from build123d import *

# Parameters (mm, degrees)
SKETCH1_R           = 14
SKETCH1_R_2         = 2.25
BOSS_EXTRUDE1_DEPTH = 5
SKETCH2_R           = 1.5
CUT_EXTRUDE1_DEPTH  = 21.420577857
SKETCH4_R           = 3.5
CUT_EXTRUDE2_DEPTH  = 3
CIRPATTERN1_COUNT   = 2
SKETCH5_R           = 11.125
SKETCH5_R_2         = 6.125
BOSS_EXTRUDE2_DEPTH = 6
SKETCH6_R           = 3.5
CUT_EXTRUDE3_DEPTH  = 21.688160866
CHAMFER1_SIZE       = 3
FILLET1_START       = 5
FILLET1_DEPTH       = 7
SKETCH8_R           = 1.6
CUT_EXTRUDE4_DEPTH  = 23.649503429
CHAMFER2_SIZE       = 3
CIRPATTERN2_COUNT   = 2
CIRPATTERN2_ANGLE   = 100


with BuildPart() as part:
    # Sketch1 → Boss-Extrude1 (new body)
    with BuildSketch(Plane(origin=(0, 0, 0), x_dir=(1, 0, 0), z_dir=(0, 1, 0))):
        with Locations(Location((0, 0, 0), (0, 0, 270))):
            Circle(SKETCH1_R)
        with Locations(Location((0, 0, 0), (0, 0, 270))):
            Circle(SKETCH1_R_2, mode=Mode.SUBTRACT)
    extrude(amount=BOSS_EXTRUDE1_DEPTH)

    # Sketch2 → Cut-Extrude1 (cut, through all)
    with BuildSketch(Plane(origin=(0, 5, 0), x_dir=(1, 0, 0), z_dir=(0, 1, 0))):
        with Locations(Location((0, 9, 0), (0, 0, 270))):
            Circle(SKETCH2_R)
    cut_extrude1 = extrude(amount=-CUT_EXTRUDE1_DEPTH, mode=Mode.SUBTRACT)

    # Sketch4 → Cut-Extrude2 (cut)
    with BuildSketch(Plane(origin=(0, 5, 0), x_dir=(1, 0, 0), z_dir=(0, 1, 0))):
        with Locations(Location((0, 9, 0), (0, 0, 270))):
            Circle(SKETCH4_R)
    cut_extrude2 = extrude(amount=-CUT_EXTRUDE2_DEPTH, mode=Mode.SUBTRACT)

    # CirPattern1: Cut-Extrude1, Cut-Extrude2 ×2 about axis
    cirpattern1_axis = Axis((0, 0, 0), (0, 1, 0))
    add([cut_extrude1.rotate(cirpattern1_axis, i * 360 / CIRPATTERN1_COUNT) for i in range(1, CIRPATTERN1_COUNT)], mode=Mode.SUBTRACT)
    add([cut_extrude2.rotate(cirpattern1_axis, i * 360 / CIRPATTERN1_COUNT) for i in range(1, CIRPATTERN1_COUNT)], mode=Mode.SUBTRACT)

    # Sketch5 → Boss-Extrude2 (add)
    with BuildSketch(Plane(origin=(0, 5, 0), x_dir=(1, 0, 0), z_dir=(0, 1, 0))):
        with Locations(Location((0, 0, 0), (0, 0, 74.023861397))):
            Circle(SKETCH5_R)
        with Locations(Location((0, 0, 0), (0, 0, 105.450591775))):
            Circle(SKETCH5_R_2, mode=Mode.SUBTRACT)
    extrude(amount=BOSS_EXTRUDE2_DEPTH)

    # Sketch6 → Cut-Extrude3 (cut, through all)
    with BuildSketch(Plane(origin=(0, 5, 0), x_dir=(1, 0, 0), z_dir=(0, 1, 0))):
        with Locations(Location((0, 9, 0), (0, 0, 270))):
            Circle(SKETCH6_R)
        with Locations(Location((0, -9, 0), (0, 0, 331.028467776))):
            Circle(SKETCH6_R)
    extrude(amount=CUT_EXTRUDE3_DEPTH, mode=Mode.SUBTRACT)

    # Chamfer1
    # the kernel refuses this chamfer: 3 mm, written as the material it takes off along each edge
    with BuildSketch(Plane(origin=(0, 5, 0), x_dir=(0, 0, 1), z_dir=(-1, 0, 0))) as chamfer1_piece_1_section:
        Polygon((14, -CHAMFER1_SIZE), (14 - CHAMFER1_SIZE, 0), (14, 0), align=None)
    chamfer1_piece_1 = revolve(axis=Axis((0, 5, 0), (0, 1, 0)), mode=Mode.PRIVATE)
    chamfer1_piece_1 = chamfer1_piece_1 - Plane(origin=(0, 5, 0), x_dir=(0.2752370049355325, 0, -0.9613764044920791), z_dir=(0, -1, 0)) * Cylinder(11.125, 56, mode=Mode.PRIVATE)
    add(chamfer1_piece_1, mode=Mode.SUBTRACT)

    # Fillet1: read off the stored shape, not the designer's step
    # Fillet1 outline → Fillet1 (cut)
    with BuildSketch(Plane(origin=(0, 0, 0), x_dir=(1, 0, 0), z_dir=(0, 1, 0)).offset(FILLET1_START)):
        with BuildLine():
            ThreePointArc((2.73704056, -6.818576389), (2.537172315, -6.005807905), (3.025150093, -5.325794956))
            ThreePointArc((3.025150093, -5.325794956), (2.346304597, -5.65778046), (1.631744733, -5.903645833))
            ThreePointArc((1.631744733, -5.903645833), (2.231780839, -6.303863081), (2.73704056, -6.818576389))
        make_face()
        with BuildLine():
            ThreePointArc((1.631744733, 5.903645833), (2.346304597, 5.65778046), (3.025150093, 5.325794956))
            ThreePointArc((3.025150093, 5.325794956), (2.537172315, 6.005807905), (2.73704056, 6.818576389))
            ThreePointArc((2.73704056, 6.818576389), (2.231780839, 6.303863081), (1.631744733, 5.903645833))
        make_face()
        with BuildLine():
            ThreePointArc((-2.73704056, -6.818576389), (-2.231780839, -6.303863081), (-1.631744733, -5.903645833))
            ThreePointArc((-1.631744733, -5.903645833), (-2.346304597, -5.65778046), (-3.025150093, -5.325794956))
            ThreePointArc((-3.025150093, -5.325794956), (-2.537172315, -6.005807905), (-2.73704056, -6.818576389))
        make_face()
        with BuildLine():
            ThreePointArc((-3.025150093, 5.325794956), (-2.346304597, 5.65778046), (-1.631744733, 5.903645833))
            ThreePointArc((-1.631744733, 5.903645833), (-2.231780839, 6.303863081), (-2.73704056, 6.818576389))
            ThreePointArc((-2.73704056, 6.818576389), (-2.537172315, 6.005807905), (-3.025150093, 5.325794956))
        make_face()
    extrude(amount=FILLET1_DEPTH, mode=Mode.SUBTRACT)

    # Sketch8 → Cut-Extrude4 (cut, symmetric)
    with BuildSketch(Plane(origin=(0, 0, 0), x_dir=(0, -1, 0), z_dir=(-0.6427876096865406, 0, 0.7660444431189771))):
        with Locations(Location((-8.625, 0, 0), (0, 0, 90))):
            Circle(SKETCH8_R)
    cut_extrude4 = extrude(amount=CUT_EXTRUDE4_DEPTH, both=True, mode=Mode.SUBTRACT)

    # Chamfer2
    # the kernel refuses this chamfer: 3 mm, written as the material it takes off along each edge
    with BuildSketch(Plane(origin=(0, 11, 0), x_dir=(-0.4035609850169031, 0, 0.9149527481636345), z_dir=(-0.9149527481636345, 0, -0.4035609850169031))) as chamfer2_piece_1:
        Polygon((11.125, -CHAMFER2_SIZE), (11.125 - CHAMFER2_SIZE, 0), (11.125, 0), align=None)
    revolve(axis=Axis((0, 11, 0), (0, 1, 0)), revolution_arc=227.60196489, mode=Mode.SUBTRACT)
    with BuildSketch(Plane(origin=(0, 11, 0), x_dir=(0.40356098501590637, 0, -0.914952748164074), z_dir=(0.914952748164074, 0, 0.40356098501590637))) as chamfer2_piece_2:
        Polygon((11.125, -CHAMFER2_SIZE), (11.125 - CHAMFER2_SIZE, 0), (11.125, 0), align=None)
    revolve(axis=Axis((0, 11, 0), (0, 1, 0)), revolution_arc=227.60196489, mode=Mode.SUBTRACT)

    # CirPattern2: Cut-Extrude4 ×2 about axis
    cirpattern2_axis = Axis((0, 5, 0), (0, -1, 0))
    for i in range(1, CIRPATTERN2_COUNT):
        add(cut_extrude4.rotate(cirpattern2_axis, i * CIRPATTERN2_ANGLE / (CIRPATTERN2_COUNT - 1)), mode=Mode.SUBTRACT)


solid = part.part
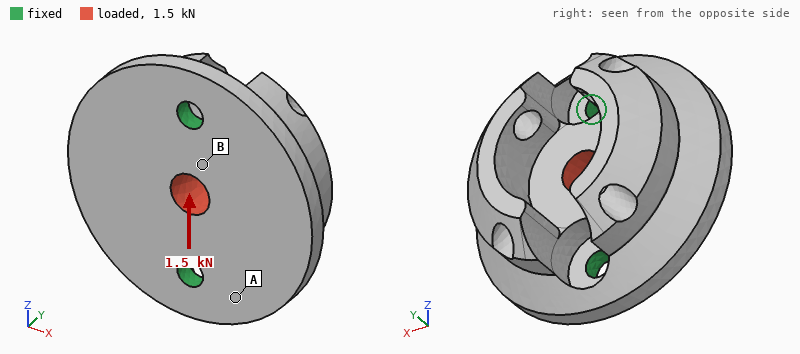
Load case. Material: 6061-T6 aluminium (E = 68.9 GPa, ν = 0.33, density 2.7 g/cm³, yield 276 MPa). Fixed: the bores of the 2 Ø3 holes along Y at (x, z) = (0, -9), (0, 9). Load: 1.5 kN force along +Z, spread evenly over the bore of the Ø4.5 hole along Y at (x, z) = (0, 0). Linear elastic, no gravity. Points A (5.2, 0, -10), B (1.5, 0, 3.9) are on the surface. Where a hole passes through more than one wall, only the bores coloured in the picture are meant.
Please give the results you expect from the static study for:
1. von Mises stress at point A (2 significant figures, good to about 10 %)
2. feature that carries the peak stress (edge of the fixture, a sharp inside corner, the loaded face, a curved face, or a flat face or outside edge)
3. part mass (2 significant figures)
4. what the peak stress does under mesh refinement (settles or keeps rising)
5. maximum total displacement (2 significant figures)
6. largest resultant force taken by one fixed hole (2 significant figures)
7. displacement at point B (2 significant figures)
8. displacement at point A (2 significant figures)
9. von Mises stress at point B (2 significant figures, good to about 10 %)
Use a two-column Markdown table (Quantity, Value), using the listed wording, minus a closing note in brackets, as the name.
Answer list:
| Quantity | Value |
|---|---|
| von Mises stress at point A | 11 MPa |
| feature that carries the peak stress | edge of the fixture |
| part mass | 8.8 g |
| what the peak stress does under mesh refinement | keeps rising |
| maximum total displacement | 4.6 µm |
| largest resultant force taken by one fixed hole | 760 N |
| displacement at point B | 2.4 µm |
| displacement at point A | 1.9 µm |
| von Mises stress at point B | 30 MPa |
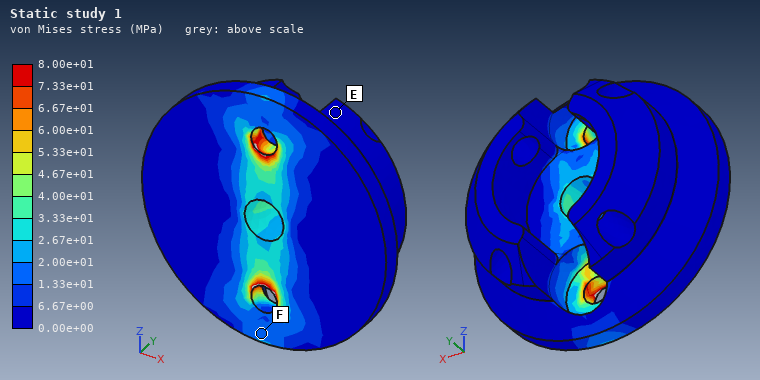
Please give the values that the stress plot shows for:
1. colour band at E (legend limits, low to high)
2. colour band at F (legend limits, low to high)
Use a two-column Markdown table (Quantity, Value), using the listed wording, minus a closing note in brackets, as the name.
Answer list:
| Quantity | Value |
|---|---|
| colour band at E | 0.00e+00 to 6.67e+00 MPa |
| colour band at F | 1.33e+01 to 2.00e+01 MPa |
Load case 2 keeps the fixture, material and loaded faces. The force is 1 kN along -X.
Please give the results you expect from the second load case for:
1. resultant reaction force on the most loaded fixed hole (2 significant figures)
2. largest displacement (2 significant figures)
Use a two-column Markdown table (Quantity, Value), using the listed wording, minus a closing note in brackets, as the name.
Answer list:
| Quantity | Value |
|---|---|
| resultant reaction force on the most loaded fixed hole | 500 N |
| largest displacement | 19 µm |
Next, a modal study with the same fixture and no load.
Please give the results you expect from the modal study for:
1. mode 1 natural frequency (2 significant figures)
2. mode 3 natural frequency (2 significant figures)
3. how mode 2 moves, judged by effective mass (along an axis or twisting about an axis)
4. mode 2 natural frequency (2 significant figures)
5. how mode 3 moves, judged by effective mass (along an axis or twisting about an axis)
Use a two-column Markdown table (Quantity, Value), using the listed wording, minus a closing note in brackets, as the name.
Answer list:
| Quantity | Value |
|---|---|
| mode 1 natural frequency | 7500 Hz |
| mode 3 natural frequency | 30 kHz |
| how mode 2 moves, judged by effective mass | along Y |
| mode 2 natural frequency | 16 kHz |
| how mode 3 moves, judged by effective mass | along Z |
